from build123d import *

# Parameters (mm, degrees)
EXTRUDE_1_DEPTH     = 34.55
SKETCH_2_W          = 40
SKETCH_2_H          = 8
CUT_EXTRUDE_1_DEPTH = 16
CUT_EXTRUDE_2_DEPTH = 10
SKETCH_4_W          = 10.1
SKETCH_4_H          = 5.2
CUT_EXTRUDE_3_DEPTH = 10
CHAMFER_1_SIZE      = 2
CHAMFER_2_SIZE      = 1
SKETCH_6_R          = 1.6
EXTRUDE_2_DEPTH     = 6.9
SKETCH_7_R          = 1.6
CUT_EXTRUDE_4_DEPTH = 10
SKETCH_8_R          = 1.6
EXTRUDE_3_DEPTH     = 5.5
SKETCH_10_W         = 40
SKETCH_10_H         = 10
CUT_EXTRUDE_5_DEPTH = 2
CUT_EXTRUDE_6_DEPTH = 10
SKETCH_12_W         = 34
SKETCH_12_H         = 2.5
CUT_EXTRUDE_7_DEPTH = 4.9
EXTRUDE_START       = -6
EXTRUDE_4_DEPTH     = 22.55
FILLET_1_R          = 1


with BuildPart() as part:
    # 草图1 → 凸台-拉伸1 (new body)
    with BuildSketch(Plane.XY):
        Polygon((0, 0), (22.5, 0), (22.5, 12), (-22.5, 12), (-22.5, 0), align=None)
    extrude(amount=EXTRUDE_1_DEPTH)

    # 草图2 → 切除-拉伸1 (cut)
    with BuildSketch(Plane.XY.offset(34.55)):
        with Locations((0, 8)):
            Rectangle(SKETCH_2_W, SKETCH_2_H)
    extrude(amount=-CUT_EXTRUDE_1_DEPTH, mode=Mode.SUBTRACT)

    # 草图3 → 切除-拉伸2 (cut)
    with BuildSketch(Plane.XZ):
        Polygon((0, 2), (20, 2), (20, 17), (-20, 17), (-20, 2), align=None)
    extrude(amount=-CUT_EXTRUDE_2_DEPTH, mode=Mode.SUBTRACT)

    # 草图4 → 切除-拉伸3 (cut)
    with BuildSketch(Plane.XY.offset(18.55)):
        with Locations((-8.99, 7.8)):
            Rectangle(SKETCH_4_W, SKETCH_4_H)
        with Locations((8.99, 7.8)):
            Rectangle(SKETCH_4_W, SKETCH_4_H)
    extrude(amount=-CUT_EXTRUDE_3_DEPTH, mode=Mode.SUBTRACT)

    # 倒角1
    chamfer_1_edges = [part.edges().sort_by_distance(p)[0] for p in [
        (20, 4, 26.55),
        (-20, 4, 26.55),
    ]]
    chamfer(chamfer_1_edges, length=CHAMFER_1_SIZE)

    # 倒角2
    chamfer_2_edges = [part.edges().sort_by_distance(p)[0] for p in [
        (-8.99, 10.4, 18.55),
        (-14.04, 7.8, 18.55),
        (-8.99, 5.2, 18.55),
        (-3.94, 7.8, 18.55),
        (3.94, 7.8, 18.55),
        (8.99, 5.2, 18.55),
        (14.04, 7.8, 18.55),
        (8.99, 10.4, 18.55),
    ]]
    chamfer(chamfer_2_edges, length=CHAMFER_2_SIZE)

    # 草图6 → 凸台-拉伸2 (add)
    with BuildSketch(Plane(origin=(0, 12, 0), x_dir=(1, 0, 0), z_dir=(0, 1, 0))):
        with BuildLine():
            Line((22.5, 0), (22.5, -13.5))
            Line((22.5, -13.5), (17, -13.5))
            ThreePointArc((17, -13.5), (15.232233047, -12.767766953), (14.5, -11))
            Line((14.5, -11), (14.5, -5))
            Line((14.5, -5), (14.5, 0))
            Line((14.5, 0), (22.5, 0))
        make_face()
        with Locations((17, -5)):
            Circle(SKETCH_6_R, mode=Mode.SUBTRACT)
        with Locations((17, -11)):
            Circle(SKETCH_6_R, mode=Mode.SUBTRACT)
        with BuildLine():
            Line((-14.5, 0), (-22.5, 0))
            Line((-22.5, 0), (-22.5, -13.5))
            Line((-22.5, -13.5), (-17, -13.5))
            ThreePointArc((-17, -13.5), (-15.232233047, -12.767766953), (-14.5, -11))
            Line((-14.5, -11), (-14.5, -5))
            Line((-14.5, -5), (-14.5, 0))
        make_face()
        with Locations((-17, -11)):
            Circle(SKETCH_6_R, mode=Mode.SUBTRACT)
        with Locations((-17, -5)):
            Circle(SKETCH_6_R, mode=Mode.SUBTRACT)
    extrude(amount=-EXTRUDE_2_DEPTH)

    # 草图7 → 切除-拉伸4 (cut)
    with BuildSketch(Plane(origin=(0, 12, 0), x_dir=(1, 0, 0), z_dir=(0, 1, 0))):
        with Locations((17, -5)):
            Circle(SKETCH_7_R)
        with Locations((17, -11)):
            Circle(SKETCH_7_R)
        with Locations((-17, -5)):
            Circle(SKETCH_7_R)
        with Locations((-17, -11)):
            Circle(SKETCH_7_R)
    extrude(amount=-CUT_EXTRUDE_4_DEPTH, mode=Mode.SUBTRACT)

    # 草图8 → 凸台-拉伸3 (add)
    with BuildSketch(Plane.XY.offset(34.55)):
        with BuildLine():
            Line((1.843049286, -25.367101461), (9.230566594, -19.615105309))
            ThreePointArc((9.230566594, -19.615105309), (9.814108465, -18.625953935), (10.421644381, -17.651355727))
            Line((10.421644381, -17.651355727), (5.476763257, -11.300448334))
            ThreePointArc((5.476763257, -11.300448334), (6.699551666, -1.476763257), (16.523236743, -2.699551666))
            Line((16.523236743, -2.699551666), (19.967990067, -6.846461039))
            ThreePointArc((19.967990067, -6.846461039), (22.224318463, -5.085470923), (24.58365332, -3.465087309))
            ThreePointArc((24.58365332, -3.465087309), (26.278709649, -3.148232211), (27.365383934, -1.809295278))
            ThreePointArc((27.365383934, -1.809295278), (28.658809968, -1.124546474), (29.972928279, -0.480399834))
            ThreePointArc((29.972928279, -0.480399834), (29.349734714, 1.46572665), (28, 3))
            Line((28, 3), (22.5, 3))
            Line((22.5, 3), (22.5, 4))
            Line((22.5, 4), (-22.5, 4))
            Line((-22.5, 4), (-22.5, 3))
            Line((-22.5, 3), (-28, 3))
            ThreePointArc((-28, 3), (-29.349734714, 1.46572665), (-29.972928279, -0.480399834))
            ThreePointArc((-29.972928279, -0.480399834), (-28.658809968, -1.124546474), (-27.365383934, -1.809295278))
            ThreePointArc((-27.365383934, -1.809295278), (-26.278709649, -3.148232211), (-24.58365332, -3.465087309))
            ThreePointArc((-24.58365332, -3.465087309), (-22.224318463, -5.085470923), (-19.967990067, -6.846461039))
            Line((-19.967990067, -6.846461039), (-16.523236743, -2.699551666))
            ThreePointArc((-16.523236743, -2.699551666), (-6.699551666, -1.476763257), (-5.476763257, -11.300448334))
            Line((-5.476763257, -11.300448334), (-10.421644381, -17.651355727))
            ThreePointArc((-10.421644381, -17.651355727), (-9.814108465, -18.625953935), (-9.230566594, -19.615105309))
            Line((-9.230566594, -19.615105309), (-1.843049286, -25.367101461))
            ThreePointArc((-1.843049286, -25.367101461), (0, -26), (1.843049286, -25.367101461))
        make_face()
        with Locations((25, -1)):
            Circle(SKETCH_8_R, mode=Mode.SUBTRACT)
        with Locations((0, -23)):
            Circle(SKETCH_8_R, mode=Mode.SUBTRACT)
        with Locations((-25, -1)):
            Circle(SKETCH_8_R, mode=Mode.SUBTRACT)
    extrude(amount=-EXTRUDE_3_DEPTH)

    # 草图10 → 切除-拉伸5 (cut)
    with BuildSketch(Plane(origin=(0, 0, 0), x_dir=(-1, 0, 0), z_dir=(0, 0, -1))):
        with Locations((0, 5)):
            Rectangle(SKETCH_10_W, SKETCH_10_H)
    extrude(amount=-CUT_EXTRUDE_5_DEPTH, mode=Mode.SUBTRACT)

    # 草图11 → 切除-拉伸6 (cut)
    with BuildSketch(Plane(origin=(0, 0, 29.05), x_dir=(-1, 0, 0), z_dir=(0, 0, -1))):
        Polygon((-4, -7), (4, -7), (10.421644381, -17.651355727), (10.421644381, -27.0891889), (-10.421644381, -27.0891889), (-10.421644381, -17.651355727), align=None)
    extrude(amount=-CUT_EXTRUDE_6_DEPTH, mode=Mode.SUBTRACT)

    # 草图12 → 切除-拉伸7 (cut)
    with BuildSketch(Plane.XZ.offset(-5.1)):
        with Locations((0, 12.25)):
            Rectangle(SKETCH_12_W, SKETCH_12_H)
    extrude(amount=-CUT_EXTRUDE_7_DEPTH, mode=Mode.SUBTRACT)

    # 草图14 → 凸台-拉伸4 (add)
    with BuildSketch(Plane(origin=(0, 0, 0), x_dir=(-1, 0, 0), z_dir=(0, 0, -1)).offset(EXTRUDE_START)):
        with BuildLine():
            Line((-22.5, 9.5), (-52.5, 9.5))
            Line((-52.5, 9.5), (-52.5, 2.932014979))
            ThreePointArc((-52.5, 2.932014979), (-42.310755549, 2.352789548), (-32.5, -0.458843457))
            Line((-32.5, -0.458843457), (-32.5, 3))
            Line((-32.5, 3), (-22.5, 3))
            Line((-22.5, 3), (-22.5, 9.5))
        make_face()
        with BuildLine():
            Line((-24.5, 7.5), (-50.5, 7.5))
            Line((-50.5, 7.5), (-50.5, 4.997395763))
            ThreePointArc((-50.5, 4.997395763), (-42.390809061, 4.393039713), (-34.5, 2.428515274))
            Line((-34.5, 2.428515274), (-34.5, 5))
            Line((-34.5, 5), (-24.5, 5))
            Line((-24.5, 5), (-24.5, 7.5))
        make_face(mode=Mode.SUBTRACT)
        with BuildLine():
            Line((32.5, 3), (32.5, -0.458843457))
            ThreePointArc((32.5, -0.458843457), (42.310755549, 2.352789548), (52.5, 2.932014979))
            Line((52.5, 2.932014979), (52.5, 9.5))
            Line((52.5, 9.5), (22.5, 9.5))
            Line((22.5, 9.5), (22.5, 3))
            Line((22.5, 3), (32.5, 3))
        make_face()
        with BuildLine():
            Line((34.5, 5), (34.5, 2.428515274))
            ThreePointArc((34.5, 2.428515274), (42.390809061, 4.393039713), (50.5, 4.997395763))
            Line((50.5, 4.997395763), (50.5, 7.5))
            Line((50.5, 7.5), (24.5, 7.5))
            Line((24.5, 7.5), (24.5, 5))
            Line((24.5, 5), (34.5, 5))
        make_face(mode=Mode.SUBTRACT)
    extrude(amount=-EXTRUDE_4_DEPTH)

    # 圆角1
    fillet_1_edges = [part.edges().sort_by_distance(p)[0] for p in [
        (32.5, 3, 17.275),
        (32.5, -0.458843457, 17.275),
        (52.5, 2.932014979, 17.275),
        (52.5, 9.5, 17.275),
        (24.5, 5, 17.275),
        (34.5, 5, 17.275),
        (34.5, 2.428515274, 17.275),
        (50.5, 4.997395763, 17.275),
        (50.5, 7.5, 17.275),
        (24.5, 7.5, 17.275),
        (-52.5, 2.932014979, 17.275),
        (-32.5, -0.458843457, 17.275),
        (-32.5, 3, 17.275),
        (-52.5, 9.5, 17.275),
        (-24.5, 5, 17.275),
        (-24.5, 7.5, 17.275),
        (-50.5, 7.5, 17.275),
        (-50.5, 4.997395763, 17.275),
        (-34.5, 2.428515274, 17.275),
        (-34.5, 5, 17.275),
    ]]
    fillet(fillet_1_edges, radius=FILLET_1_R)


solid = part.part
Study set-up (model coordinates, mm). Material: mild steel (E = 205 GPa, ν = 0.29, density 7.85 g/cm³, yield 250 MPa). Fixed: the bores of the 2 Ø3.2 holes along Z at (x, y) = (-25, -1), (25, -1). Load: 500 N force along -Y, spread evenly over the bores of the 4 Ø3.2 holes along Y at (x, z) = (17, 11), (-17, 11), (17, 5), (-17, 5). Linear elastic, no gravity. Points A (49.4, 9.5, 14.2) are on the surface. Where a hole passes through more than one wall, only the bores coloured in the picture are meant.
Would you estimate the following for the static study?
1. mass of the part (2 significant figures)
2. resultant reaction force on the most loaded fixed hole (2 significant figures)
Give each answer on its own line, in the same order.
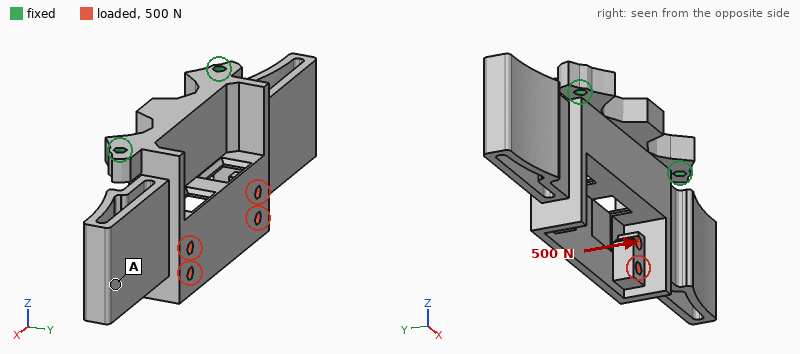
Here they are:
110 g
280 N
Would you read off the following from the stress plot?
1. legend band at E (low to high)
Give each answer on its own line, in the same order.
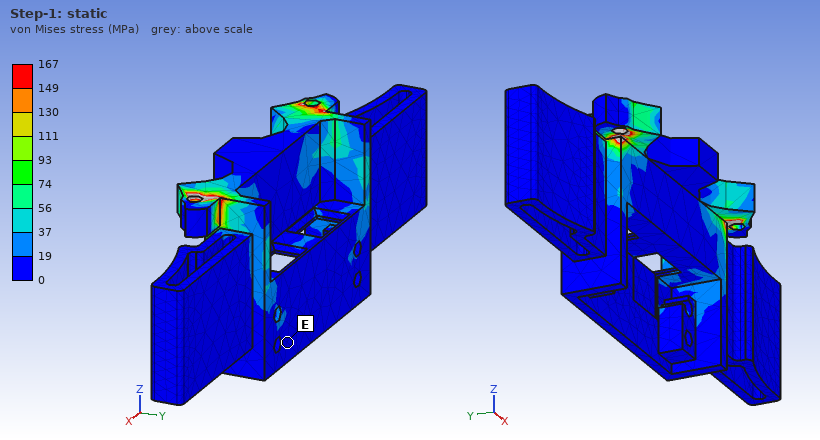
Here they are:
0 to 19 MPa
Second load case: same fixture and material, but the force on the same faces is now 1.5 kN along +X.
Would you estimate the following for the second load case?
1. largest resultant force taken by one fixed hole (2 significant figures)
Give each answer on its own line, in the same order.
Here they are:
1.1 kN
